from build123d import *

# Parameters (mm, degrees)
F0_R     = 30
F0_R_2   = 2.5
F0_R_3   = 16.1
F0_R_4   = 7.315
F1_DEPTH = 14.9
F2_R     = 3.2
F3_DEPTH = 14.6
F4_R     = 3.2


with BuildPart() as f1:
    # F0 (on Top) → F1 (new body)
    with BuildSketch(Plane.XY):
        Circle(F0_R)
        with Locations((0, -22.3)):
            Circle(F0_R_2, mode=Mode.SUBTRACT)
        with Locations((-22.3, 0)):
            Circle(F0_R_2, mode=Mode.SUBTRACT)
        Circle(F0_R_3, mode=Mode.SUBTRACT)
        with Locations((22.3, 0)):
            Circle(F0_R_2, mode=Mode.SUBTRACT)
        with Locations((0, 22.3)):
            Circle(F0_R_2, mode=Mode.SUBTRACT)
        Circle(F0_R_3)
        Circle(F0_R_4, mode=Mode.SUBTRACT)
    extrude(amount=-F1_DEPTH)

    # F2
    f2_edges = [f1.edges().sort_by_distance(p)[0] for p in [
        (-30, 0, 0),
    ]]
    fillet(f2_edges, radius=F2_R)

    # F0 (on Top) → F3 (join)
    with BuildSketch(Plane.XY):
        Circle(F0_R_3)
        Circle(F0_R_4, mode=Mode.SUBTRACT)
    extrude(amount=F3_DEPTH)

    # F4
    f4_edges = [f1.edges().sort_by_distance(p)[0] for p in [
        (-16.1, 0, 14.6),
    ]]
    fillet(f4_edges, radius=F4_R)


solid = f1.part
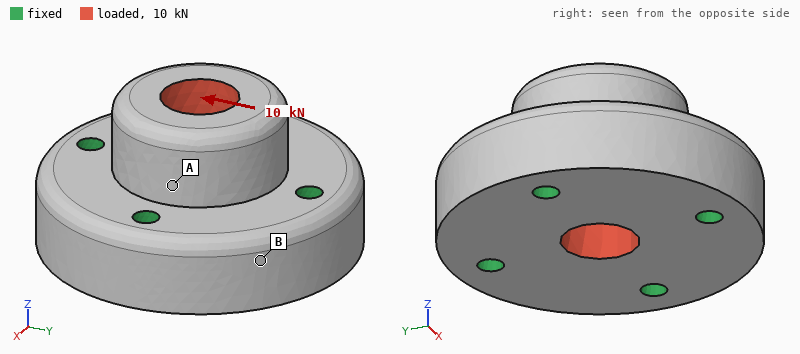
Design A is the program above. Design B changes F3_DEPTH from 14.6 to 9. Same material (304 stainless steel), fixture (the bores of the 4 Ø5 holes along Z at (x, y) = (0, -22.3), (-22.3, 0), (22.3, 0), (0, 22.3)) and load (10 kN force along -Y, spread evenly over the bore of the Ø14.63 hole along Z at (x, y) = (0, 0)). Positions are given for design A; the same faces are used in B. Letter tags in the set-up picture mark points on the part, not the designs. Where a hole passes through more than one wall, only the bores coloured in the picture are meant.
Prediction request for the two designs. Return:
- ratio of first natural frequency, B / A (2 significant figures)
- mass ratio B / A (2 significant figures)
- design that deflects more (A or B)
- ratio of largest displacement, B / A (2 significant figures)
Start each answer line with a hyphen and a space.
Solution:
- 1.2
- 0.92
- A
- 0.66
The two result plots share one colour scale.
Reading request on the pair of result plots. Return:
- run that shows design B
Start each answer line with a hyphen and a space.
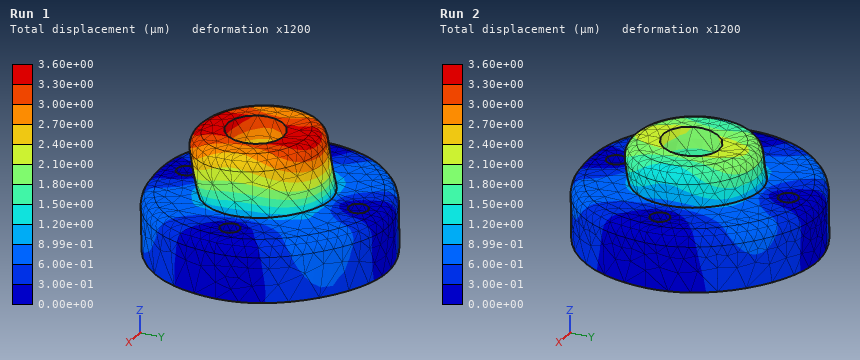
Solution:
- Run 2
